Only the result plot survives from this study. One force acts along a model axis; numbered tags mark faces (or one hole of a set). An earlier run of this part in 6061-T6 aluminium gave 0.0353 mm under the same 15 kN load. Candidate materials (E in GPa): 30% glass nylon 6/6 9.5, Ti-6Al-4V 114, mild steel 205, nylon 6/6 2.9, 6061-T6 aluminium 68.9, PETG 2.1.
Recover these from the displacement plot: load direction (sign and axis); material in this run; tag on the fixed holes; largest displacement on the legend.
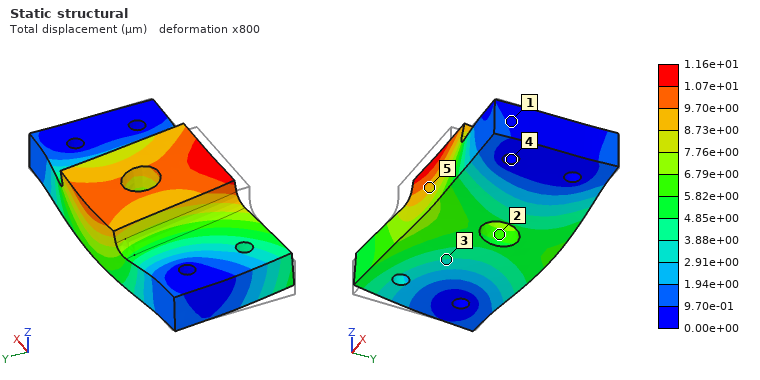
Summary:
+Y
mild steel
4
1.16e+01 µm
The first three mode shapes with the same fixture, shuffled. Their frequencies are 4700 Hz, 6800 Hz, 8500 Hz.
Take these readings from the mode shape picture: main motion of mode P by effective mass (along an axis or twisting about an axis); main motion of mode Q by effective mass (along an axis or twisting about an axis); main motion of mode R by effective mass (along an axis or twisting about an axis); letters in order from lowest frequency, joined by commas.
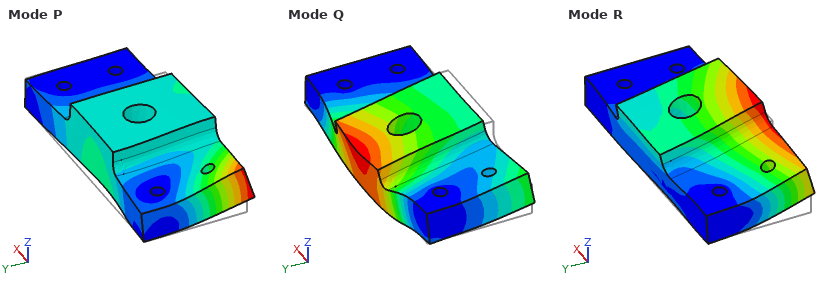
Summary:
along Y
along Z
along Z
R, Q, P
